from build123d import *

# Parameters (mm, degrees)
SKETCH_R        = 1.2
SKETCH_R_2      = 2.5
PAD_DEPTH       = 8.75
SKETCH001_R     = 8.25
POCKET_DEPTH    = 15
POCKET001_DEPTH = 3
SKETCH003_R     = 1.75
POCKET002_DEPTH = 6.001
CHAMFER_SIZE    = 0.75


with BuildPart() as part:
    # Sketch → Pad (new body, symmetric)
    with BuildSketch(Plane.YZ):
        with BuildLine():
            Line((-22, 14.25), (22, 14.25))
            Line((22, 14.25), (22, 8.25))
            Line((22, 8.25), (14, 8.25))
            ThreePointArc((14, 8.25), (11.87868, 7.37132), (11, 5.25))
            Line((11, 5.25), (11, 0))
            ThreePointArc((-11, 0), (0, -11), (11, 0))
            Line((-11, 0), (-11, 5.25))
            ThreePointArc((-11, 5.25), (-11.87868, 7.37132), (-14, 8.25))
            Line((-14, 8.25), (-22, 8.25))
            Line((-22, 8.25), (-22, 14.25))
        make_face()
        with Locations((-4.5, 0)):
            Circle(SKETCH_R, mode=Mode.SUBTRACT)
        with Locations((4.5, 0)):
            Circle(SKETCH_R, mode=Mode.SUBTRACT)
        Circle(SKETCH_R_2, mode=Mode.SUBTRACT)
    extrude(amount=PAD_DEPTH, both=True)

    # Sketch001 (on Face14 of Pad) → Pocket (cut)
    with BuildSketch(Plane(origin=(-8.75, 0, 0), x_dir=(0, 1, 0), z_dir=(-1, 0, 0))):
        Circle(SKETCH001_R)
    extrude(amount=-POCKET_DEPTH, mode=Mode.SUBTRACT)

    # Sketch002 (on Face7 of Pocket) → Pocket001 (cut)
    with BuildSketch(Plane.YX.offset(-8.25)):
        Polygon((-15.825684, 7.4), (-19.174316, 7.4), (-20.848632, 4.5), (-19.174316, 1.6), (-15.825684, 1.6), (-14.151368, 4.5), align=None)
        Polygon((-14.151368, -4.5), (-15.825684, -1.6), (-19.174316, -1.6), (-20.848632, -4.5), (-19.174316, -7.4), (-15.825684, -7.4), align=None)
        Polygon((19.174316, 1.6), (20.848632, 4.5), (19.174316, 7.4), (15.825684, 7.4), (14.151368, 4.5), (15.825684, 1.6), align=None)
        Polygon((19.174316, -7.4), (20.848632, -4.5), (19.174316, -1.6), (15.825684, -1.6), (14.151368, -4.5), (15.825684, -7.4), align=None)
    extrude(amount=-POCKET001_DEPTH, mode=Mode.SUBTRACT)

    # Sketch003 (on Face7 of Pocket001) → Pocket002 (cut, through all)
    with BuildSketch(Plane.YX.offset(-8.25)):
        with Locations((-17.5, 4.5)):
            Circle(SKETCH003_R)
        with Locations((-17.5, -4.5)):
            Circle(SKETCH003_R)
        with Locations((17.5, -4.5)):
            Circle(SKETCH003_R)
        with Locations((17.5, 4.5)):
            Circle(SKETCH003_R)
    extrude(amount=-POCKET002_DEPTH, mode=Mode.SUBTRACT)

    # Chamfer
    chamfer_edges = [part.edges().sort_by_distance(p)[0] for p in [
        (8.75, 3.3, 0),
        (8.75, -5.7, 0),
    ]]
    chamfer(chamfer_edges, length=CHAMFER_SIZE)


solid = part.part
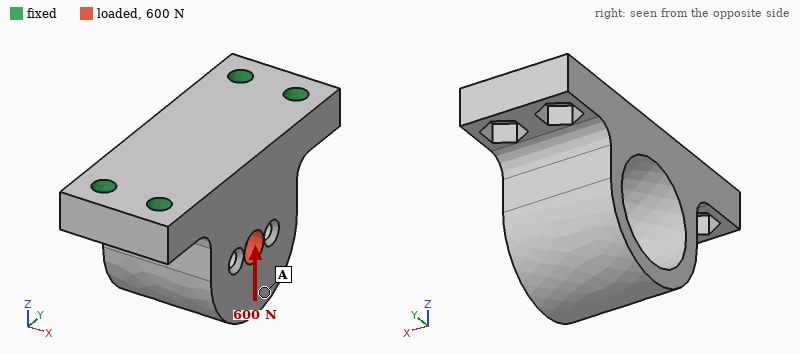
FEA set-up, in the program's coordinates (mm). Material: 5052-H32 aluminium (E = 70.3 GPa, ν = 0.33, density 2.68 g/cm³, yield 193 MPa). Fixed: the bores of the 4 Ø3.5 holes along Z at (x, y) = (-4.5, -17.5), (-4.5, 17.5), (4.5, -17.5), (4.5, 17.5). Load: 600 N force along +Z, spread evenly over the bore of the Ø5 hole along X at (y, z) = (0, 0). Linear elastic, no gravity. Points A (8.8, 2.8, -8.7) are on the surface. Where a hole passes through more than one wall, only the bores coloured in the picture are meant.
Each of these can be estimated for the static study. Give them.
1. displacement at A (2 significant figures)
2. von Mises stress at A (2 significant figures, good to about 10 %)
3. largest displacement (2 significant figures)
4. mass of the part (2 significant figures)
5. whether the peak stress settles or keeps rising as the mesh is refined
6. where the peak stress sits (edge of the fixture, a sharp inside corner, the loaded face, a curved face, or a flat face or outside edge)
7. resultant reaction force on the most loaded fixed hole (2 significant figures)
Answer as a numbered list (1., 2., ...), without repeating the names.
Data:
1. 13 µm
2. 7.3 MPa
3. 14 µm
4. 20 g
5. keeps rising
6. edge of the fixture
7. 420 N
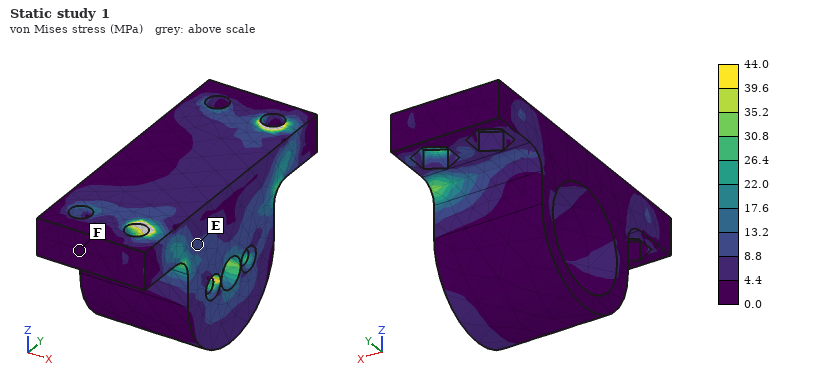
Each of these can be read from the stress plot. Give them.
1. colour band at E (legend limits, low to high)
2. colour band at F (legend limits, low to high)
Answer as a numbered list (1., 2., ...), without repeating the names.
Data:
1. 8.8 to 13.2 MPa
2. 0.0 to 4.4 MPa
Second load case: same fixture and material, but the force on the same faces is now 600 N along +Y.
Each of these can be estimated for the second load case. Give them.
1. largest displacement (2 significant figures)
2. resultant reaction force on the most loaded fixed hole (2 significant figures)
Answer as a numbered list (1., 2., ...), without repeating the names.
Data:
1. 7.4 µm
2. 230 N
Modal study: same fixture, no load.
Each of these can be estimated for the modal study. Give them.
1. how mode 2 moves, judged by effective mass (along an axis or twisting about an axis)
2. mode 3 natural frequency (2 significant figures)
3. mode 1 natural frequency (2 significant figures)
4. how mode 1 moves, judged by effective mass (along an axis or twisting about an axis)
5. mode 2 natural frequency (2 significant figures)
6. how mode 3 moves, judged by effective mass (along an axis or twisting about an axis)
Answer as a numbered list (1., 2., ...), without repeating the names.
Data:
1. along Y
2. 18 kHz
3. 10000 Hz
4. along X
5. 15 kHz
6. along Z
